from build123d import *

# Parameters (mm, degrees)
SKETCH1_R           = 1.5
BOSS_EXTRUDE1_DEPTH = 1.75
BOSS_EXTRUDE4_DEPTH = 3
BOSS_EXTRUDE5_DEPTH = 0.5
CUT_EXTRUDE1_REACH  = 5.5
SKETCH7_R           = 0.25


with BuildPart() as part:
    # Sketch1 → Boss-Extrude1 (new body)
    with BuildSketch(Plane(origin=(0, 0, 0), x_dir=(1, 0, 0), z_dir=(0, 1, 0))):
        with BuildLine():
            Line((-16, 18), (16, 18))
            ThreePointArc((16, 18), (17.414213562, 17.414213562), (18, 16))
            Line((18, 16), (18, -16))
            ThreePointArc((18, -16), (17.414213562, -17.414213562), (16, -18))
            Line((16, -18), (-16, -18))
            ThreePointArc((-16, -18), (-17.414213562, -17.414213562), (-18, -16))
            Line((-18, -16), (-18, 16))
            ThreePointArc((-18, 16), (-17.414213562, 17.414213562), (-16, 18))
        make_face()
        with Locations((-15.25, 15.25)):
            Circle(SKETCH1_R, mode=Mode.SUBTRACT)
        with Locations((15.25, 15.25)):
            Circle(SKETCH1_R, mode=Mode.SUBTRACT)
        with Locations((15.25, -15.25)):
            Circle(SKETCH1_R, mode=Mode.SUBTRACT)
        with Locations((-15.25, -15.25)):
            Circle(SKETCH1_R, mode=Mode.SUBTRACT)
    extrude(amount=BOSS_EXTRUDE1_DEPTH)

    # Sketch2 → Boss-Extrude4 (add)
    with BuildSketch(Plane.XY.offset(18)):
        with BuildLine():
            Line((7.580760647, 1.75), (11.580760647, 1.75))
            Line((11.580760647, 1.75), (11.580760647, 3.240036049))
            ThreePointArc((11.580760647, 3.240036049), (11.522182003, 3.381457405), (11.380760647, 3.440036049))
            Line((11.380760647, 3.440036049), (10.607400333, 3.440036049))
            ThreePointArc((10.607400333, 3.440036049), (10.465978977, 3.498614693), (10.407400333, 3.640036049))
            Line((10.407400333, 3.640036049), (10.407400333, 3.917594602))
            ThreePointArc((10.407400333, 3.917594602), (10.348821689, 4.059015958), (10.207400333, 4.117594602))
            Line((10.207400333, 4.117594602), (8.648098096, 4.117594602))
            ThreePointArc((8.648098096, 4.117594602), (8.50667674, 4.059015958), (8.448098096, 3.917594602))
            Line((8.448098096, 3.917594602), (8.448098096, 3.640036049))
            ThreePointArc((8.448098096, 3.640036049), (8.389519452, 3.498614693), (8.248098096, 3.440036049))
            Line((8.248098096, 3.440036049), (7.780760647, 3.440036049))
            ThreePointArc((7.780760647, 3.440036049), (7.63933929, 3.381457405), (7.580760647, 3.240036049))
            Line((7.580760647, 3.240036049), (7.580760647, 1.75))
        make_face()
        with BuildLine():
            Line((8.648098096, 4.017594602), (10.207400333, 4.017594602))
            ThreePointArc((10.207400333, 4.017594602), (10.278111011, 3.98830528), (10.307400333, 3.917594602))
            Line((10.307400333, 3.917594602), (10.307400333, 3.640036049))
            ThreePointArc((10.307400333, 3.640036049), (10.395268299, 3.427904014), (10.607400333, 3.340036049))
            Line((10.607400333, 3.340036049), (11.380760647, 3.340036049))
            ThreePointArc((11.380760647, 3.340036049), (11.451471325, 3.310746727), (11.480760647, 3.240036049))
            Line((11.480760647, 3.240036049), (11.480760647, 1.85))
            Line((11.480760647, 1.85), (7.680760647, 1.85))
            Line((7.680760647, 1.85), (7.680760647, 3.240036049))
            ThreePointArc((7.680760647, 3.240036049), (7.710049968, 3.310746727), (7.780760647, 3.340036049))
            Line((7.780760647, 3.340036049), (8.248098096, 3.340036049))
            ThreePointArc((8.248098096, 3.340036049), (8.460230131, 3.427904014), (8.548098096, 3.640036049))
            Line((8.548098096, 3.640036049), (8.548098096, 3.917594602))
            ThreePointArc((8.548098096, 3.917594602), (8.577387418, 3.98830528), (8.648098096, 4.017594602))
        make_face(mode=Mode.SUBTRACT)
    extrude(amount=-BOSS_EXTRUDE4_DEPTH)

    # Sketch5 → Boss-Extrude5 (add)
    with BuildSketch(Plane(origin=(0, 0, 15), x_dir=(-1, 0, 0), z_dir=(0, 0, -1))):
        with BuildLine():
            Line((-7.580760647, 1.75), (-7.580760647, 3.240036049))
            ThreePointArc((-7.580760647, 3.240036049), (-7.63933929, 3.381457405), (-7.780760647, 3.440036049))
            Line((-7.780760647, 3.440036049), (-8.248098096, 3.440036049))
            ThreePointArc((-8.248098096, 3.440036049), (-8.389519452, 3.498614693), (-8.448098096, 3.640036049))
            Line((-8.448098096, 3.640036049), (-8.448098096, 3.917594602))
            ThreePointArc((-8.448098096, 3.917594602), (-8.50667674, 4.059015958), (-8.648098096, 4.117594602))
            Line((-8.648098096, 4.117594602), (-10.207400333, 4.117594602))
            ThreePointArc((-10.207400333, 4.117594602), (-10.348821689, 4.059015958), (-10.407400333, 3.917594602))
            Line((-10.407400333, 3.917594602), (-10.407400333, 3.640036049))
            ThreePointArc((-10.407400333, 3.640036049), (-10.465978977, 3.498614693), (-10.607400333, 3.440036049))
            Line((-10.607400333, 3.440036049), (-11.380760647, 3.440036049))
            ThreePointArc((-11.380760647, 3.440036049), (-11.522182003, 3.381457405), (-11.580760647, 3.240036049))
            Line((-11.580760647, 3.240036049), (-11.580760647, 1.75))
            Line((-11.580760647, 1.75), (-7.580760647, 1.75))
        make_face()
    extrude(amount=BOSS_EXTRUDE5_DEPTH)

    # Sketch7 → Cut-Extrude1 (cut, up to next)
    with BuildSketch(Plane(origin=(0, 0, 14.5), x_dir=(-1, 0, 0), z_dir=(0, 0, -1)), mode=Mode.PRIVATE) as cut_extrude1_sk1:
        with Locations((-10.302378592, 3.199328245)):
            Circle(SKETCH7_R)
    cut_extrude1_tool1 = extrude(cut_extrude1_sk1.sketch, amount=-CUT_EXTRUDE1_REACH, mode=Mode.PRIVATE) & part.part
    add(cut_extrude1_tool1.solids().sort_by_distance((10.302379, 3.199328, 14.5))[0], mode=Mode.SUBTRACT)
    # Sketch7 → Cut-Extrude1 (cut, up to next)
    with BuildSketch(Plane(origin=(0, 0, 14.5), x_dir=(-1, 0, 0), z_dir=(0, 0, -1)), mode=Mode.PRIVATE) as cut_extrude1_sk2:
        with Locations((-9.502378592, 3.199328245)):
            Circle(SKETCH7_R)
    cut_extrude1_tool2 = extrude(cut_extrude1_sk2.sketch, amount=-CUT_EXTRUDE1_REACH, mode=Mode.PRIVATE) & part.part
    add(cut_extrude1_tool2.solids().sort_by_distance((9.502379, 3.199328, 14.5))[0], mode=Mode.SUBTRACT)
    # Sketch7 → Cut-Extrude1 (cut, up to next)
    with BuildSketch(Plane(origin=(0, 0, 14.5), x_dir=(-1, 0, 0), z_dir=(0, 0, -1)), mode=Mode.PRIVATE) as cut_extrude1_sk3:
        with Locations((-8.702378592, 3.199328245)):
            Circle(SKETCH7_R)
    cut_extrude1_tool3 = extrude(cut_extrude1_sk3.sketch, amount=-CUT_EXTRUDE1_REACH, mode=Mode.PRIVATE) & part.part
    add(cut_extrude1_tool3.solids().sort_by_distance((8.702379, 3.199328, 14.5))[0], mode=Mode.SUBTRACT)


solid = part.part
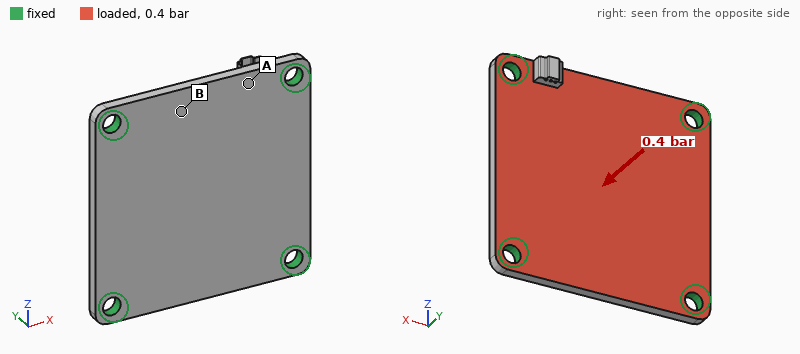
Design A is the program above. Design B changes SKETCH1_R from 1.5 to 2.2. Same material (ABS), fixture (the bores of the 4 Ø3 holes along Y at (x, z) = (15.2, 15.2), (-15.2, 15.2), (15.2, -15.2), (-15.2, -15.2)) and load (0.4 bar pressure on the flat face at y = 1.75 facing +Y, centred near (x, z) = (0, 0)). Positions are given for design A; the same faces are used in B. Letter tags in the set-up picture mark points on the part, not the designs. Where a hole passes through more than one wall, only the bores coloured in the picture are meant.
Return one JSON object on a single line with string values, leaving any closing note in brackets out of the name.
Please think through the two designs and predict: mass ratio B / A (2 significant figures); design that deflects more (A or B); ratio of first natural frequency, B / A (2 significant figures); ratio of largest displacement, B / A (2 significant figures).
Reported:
{"mass ratio B / A": "0.97", "design that deflects more": "A", "ratio of first natural frequency, B / A": "1.1", "ratio of largest displacement, B / A": "0.82"}
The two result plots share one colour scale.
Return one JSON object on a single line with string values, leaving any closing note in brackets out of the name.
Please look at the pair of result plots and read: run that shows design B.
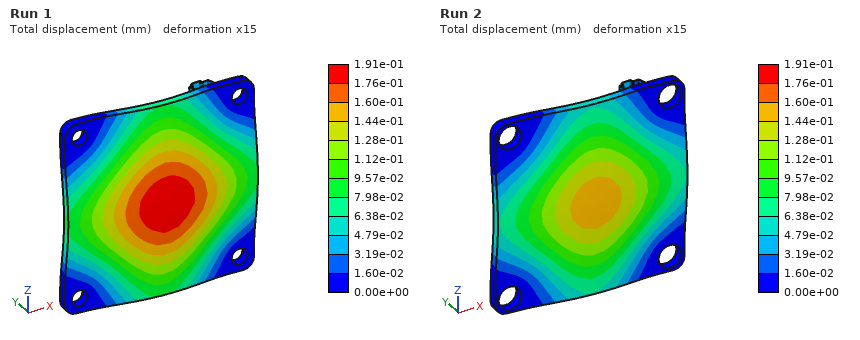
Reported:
{"run that shows design B": "Run 2"}
